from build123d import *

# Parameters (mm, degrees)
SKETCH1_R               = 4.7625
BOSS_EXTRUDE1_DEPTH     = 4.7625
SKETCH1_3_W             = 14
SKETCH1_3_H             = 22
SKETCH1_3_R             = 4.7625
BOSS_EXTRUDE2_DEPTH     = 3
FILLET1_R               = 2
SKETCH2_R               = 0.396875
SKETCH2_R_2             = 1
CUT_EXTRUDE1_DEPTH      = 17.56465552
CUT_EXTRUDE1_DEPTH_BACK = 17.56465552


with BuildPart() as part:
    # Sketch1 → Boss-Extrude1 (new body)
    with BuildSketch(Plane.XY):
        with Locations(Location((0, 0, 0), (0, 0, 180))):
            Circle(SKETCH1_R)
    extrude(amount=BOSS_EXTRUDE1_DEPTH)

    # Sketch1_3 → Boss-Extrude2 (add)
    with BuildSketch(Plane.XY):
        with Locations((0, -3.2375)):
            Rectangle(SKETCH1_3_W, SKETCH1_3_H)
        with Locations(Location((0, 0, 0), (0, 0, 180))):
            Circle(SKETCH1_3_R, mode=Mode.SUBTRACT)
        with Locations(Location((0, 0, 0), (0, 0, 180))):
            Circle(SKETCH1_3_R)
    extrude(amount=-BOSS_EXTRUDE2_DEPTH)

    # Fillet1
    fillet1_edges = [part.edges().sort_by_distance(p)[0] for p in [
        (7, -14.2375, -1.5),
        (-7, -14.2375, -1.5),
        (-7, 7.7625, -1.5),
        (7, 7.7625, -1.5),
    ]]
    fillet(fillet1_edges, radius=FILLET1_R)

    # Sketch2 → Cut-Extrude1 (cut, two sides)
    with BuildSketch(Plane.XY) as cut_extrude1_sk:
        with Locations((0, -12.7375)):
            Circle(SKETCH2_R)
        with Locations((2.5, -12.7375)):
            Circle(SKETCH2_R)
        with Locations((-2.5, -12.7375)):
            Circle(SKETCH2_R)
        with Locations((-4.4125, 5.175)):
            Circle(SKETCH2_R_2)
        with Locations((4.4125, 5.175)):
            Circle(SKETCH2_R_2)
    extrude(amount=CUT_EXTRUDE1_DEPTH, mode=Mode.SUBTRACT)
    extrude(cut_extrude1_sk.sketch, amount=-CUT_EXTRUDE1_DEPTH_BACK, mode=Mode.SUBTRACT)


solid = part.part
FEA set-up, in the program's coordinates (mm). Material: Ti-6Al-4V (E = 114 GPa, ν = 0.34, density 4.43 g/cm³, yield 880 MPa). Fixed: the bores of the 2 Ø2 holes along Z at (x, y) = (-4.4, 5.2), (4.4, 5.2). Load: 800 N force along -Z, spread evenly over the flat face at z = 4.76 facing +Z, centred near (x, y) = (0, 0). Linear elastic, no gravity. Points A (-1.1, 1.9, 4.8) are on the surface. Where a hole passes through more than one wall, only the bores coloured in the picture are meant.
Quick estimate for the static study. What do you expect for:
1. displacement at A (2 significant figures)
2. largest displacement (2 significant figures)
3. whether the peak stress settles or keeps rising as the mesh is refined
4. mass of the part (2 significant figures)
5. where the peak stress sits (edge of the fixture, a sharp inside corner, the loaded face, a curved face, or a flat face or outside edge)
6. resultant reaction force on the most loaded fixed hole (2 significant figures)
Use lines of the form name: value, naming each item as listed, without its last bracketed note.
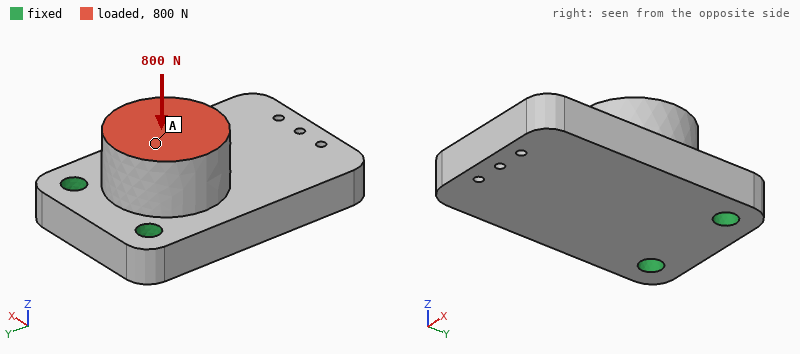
displacement at A: 18 µm
largest displacement: 51 µm
whether the peak stress settles or keeps rising as the mesh is refined: keeps rising
mass of the part: 5.4 g
where the peak stress sits: edge of the fixture
resultant reaction force on the most loaded fixed hole: 400 N
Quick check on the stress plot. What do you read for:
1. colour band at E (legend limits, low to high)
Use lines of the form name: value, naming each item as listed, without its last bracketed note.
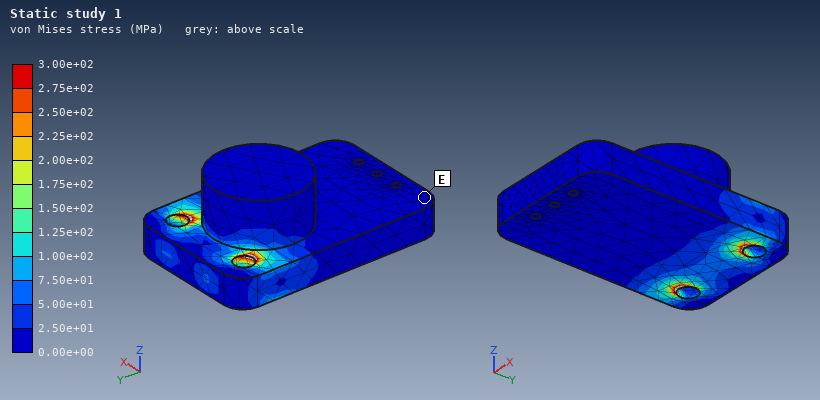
colour band at E: 0.00e+00 to 2.50e+01 MPa
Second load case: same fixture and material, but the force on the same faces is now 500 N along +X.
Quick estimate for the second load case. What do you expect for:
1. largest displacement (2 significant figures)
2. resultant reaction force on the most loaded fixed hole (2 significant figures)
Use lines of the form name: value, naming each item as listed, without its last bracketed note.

largest displacement: 7.1 µm
resultant reaction force on the most loaded fixed hole: 490 N
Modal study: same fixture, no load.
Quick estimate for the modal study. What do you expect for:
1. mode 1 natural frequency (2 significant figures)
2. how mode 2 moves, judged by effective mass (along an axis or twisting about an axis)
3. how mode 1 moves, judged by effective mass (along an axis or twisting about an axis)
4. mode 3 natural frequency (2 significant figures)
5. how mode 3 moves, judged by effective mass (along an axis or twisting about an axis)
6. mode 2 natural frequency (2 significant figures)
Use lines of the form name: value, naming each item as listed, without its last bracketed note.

mode 1 natural frequency: 7700 Hz
how mode 2 moves, judged by effective mass: along X
how mode 1 moves, judged by effective mass: along Z
mode 3 natural frequency: 25 kHz
how mode 3 moves, judged by effective mass: along X
mode 2 natural frequency: 23 kHz
